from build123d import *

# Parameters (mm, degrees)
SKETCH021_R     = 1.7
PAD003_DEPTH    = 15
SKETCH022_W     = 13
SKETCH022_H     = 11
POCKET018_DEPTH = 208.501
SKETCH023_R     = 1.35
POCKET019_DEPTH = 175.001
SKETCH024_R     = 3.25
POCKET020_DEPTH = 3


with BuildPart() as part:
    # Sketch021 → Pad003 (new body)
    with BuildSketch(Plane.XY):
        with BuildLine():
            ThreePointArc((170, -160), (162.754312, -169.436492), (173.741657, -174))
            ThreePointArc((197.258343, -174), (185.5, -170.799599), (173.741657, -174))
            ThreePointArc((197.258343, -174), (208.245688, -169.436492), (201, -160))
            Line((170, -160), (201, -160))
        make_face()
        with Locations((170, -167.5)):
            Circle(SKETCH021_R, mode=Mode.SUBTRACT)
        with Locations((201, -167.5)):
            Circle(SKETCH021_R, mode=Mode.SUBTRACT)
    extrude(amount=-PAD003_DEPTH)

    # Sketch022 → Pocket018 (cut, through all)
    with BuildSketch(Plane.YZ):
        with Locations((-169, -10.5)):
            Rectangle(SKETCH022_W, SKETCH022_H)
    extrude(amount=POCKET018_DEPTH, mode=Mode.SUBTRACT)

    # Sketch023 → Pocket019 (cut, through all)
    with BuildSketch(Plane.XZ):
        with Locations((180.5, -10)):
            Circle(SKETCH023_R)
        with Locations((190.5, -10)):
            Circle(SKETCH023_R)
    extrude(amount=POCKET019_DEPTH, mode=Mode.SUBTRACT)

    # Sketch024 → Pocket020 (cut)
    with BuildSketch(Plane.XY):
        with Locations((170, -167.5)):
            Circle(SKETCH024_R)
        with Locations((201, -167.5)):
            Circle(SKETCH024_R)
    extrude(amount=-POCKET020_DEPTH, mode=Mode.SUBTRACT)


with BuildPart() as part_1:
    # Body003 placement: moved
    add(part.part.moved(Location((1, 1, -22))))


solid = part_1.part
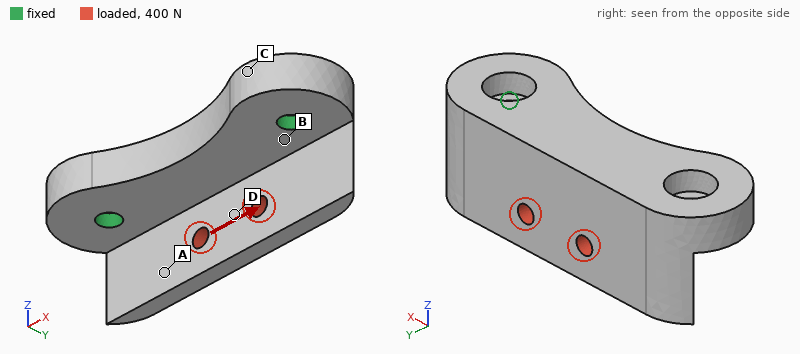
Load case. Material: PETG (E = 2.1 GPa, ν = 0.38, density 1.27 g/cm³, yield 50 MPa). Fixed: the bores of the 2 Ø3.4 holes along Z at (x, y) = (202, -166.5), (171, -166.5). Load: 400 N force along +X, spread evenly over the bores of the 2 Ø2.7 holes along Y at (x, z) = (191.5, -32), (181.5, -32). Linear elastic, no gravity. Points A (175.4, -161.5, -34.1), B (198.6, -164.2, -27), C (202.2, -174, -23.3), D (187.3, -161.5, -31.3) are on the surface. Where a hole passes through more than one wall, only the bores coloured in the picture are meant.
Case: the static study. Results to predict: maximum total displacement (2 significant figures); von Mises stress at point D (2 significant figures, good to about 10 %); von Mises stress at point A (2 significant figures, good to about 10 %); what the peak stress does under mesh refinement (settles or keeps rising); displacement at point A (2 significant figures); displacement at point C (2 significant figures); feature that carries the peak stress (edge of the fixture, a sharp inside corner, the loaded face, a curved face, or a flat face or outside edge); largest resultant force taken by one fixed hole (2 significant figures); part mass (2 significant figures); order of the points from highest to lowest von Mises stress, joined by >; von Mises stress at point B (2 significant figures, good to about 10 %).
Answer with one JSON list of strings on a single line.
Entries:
["0.26 mm", "10 MPa", "5.9 MPa", "keeps rising", "0.16 mm", "0.071 mm", "edge of the fixture", "220 N", "4.5 g", "B > D > A > C", "15 MPa"]
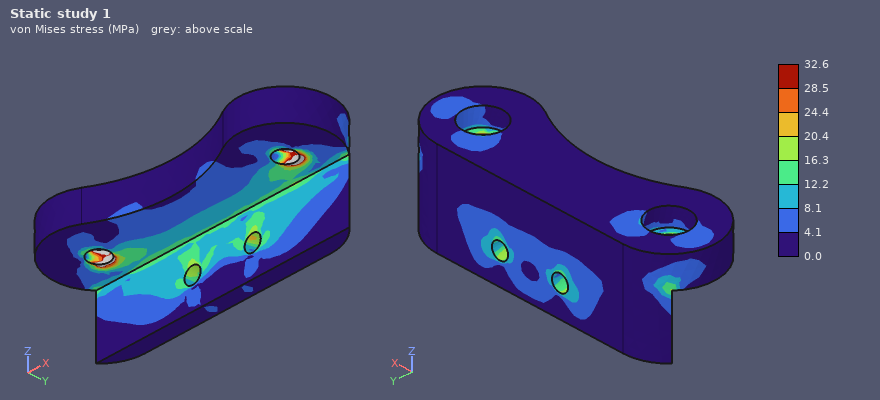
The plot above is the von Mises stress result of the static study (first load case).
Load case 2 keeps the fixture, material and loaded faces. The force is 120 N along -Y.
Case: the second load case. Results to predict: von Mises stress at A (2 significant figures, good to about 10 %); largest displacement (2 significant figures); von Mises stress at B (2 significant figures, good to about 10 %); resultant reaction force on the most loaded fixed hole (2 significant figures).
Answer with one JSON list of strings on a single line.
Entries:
["3.3 MPa", "0.60 mm", "11 MPa", "66 N"]
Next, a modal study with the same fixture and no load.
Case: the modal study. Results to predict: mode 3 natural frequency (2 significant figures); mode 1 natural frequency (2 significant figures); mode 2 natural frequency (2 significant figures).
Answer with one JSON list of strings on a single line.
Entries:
["4600 Hz", "2400 Hz", "3800 Hz"]
